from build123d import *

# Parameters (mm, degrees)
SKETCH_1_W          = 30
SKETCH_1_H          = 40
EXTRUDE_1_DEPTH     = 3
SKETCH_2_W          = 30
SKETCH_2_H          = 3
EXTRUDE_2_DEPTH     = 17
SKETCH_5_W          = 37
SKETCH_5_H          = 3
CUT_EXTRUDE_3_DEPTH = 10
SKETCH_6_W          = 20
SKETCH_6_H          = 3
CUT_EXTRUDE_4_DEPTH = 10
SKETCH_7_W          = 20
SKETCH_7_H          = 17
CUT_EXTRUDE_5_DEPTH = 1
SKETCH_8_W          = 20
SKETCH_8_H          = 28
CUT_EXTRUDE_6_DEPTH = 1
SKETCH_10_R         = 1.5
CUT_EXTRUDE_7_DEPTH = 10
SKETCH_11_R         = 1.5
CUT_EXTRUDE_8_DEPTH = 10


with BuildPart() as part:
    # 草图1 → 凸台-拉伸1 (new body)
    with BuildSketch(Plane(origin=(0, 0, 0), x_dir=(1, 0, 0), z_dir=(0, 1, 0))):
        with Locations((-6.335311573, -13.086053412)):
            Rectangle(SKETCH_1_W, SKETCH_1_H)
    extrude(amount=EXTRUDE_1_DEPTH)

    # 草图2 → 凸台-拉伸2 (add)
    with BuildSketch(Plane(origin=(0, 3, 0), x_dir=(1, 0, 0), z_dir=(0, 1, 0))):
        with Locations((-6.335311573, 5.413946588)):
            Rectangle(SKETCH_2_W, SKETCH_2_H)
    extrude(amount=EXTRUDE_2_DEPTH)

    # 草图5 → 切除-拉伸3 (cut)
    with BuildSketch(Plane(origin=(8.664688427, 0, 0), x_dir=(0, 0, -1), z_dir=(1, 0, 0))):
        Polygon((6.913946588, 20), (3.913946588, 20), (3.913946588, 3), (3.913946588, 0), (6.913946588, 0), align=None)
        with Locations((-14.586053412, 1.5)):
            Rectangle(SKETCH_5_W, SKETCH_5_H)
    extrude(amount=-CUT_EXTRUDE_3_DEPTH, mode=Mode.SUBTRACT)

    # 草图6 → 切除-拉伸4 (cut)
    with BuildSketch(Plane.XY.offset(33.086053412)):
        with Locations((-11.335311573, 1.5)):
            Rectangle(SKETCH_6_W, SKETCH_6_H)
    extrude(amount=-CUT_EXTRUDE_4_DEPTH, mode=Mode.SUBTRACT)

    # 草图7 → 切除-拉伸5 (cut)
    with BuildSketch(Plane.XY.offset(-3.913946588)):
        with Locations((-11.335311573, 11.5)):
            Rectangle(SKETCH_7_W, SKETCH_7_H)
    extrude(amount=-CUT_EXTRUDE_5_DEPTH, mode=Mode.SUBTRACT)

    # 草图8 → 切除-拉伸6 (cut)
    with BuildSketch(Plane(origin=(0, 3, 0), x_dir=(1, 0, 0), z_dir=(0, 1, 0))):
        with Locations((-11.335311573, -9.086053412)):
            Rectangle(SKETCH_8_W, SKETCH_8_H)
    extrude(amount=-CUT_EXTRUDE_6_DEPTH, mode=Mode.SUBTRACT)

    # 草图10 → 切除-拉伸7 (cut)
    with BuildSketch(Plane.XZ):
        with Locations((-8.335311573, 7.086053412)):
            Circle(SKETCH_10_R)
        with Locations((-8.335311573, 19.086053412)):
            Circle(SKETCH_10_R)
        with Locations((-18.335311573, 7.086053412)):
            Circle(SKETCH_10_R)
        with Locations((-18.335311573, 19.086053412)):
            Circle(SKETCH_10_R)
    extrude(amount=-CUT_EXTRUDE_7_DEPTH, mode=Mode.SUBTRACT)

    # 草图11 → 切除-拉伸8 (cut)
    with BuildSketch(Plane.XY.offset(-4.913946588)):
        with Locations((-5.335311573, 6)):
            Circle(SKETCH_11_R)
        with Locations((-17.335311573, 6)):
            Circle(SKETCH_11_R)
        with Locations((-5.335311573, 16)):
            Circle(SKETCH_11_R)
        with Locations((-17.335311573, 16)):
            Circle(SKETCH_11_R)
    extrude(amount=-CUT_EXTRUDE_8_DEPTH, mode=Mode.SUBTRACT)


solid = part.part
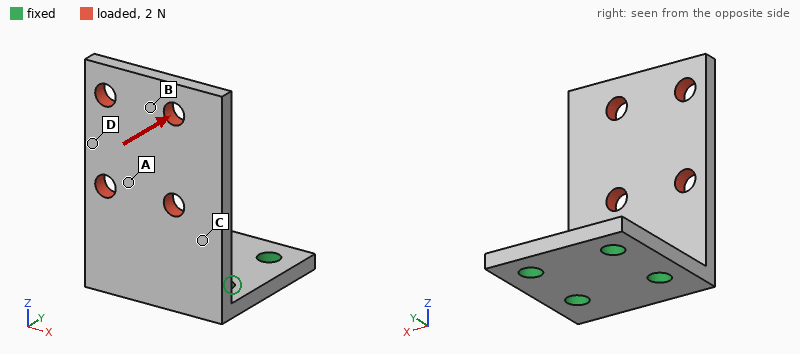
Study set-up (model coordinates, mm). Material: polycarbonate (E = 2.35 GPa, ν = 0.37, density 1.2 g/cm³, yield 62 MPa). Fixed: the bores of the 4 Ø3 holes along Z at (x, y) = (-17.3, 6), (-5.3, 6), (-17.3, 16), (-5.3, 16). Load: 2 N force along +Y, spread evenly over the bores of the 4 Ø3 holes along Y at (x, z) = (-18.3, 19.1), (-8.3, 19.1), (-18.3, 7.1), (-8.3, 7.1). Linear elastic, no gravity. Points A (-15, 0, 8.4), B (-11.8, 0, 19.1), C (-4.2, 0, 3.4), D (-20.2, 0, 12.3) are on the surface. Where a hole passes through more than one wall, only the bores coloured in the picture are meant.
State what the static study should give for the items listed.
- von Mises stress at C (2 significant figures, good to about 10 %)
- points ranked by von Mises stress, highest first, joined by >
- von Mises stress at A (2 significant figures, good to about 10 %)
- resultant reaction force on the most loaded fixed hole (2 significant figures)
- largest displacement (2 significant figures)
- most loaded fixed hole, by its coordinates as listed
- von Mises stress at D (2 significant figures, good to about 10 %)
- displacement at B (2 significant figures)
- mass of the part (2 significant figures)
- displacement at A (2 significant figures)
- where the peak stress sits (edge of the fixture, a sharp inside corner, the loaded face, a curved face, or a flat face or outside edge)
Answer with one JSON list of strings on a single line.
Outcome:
["1.5 MPa", "C > A > D > B", "1.0 MPa", "1.2 N", "0.40 mm", "(-17.3, 6)", "0.51 MPa", "0.32 mm", "2.2 g", "0.15 mm", "a flat face or outside edge"]
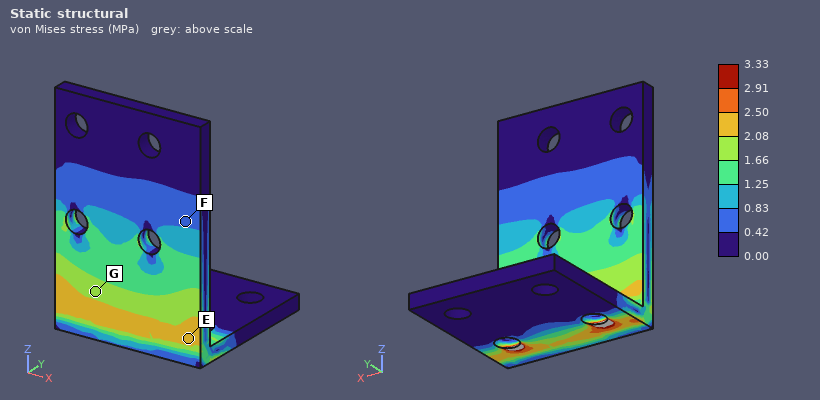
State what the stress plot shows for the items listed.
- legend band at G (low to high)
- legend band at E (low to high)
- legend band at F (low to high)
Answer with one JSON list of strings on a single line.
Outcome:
["1.66 to 2.08 MPa", "2.08 to 2.50 MPa", "0.42 to 0.83 MPa"]
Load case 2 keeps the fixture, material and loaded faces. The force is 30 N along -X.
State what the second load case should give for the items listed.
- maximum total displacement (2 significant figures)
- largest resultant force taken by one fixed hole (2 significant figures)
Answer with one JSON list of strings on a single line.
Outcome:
["0.37 mm", "46 N"]
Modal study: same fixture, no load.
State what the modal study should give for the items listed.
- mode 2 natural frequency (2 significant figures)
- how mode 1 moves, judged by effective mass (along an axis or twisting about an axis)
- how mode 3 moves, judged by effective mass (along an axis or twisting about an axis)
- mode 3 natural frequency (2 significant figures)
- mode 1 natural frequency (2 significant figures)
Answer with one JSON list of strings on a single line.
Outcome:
["1500 Hz", "along Y", "along X", "2000 Hz", "470 Hz"]
